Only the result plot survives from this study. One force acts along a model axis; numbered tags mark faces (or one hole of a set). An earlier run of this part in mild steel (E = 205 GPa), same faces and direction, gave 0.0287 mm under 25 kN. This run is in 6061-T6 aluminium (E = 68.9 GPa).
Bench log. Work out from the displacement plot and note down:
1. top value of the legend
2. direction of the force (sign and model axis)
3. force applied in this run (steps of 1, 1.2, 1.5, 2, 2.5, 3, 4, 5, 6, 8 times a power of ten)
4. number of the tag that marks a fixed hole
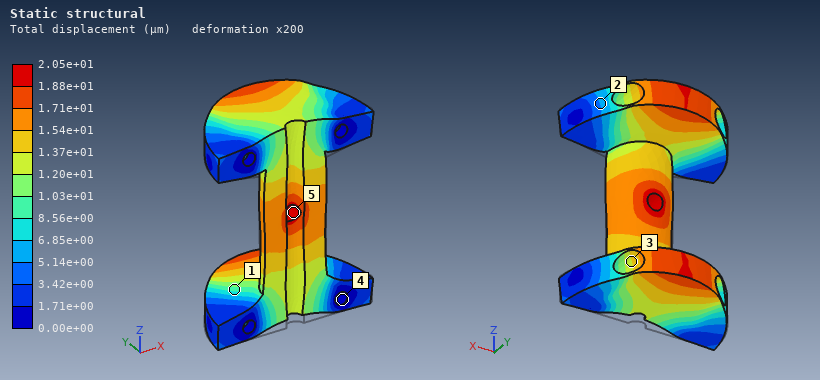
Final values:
2.05e+01 µm
+Z
6 kN
4
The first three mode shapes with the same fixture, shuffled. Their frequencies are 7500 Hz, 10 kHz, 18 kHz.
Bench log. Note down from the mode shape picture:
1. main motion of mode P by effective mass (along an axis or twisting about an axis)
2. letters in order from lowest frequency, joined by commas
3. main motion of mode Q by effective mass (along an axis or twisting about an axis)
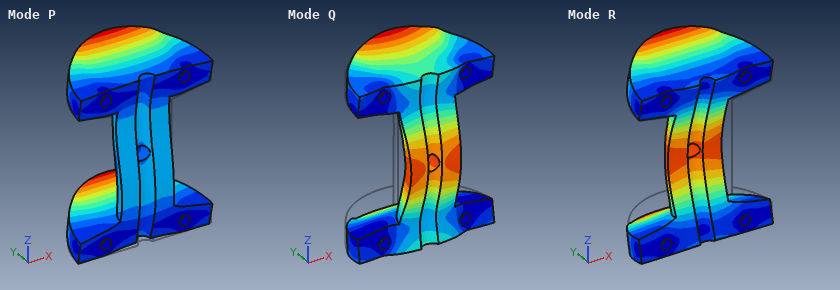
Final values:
along Z
R, P, Q
along Y
